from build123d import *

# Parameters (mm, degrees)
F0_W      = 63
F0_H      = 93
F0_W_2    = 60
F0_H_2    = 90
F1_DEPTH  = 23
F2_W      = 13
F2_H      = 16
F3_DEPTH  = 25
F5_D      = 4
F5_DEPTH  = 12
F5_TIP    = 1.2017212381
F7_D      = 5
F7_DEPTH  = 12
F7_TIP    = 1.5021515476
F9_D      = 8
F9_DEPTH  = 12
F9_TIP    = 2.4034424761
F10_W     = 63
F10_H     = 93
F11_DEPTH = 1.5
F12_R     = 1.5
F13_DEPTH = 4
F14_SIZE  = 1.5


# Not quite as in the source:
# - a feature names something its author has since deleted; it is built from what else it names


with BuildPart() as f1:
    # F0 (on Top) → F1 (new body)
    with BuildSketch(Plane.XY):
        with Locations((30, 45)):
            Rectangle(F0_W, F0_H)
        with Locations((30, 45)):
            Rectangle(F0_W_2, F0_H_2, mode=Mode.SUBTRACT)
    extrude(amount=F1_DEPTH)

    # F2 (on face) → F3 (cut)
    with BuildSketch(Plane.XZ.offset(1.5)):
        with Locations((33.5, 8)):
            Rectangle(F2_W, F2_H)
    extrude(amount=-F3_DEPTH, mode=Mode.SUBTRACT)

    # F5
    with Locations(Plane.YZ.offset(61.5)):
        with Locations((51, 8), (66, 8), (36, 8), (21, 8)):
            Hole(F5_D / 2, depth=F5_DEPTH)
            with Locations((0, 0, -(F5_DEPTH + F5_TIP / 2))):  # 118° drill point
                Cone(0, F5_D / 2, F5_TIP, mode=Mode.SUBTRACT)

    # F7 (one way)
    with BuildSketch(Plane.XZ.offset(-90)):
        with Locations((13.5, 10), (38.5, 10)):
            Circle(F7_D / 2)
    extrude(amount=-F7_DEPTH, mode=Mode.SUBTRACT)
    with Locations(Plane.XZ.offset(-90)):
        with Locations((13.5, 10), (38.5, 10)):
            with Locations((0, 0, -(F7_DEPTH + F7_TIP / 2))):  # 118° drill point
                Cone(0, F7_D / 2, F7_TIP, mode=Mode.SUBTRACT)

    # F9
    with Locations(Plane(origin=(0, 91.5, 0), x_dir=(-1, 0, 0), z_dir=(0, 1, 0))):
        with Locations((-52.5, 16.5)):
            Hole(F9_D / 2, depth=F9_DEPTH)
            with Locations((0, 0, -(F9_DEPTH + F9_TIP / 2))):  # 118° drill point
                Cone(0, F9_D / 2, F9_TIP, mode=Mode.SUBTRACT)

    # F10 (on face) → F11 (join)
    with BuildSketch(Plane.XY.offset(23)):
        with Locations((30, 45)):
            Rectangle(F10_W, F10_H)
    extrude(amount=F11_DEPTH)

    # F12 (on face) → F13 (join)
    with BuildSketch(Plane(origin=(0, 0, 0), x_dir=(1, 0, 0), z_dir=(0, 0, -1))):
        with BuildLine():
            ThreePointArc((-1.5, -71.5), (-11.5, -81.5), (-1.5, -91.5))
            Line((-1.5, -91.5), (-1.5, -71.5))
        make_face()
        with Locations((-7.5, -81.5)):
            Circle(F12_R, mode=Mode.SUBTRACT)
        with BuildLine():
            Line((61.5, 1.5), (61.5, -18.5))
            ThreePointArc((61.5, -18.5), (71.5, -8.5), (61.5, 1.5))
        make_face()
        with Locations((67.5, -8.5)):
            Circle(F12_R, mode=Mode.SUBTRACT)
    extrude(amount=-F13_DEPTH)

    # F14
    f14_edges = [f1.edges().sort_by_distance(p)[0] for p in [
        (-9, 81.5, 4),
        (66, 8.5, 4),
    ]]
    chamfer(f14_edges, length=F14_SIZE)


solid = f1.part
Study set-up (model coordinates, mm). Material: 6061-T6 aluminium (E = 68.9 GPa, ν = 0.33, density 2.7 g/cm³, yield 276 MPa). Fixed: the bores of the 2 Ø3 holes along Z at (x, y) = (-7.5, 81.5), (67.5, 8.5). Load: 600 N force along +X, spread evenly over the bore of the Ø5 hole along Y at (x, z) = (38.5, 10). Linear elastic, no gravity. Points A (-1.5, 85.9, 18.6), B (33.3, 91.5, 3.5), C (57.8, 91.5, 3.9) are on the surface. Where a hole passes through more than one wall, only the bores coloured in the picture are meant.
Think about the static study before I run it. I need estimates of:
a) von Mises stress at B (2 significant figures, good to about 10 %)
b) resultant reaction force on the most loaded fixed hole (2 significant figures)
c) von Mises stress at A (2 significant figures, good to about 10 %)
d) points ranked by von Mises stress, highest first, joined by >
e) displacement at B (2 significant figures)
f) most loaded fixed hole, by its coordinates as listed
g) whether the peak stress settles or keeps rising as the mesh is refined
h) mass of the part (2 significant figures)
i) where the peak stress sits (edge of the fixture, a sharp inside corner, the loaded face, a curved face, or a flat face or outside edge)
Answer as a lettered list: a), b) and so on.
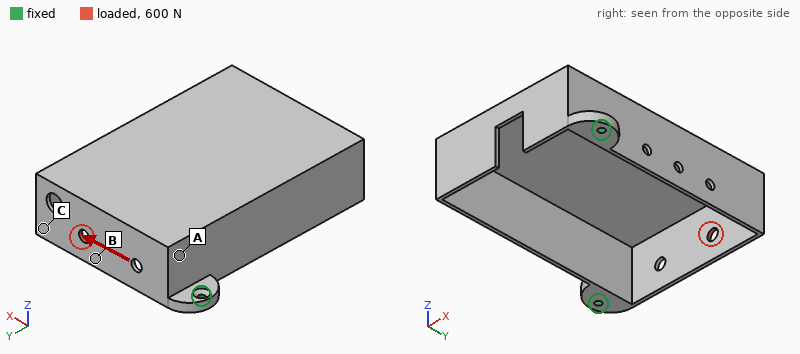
a) 27 MPa
b) 550 N
c) 14 MPa
d) B > A > C
e) 0.15 mm
f) (-7.5, 81.5)
g) keeps rising
h) 54 g
i) edge of the fixture
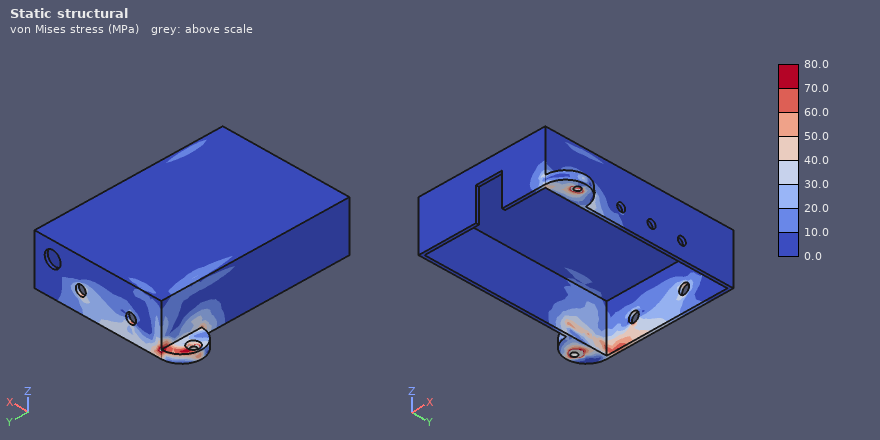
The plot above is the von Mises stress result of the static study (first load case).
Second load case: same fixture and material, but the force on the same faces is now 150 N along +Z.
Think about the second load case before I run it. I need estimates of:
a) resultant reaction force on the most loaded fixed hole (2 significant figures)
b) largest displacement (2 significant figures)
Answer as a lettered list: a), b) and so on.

a) 130 N
b) 0.45 mm
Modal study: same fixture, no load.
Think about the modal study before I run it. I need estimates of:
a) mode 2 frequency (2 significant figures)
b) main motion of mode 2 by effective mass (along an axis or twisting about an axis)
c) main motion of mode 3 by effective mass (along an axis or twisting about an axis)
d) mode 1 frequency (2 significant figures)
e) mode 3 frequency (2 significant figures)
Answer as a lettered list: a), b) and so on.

a) 1700 Hz
b) along Z
c) along X
d) 610 Hz
e) 1900 Hz
